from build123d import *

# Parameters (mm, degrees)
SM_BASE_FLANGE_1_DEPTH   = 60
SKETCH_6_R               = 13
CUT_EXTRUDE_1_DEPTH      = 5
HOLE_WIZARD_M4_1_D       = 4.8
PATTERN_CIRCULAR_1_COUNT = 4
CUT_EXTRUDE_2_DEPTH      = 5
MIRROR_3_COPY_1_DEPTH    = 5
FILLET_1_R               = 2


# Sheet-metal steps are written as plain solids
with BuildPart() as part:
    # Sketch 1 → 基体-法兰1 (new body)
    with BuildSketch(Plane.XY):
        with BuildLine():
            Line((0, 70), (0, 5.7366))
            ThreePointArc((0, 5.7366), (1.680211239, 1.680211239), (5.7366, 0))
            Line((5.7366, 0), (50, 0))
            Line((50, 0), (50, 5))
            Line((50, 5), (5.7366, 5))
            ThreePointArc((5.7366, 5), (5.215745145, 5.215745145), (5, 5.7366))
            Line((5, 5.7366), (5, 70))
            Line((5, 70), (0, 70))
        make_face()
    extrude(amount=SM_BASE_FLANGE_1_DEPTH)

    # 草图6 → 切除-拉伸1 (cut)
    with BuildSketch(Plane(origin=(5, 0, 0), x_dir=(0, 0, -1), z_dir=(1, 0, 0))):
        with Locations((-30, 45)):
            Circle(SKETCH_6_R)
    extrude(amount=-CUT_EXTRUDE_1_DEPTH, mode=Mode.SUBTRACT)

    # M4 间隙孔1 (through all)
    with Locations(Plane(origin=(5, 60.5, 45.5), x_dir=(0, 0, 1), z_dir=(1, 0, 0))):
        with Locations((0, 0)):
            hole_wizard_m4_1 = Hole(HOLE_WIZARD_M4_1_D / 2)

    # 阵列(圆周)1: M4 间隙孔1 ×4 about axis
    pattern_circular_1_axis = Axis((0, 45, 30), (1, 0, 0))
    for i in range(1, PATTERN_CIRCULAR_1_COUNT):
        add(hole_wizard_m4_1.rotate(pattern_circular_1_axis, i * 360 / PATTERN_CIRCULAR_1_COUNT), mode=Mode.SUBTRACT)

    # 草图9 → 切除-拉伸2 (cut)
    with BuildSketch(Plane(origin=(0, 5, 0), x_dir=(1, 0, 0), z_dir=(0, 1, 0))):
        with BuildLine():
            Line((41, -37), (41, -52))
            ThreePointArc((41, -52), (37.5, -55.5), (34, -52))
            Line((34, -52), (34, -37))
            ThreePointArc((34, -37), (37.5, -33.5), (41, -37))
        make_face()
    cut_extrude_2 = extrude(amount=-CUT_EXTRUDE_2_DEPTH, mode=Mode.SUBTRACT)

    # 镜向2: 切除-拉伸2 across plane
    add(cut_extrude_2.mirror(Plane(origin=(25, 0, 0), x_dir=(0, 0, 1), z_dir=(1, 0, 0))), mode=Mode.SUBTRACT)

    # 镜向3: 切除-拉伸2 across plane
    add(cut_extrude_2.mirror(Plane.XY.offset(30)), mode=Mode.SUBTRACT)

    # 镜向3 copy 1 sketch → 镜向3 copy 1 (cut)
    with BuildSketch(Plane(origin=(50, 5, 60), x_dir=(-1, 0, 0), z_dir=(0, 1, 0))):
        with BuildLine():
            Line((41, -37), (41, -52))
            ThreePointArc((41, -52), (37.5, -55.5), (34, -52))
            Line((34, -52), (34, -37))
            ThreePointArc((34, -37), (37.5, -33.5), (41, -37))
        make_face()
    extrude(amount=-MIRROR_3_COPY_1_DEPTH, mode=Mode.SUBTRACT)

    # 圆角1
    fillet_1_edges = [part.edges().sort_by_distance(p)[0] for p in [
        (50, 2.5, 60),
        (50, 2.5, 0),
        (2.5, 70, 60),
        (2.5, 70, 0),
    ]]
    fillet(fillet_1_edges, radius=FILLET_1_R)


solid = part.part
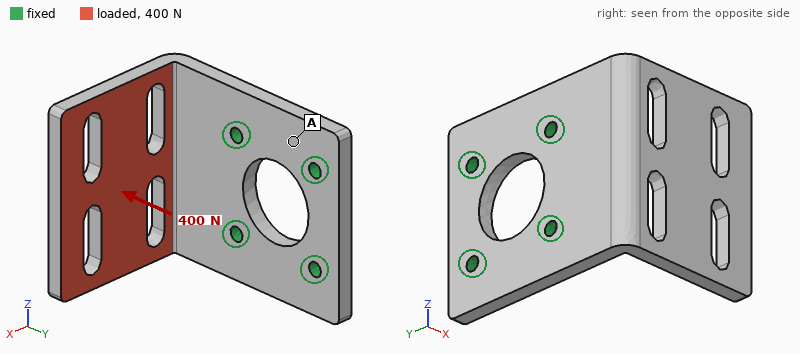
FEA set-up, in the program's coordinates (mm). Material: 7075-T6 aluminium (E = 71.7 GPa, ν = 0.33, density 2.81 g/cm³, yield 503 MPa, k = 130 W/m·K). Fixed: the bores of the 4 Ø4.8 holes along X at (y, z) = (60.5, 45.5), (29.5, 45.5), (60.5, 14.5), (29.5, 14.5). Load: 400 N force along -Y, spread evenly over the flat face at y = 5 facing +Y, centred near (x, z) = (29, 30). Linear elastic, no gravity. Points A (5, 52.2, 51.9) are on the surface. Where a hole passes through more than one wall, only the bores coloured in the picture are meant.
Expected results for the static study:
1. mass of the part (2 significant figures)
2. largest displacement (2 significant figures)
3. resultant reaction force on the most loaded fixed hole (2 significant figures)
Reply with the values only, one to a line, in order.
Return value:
79 g
0.62 mm
190 N
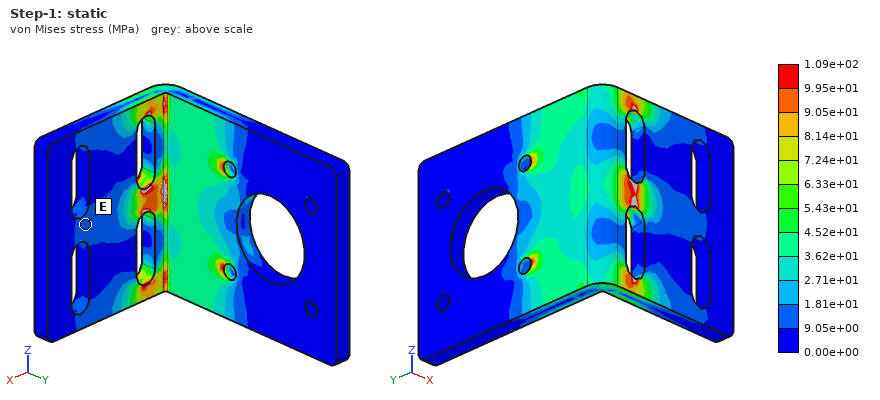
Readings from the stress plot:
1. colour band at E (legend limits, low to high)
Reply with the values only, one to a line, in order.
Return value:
9.05e+00 to 1.81e+01 MPa
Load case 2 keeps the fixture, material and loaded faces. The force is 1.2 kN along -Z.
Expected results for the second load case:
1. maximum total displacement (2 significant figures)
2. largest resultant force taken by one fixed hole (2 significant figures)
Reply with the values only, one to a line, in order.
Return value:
0.39 mm
1.2 kN
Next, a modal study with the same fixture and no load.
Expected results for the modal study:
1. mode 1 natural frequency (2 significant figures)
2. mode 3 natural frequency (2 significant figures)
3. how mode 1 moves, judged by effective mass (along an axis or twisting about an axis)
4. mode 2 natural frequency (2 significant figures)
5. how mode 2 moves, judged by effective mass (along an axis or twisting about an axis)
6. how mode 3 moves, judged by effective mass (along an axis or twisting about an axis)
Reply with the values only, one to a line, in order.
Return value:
890 Hz
2600 Hz
along Y
1800 Hz
along Z
along X
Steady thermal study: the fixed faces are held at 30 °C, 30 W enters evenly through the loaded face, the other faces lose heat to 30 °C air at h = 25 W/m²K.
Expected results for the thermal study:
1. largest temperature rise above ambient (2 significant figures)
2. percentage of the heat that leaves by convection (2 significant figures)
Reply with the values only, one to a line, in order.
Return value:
57 K
19 %
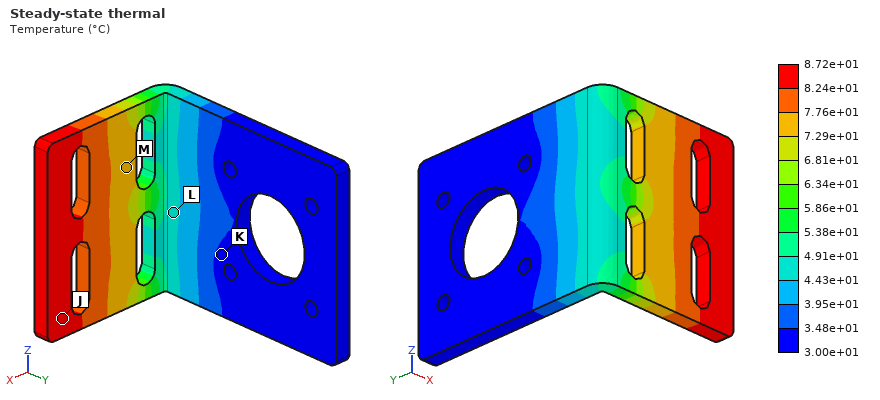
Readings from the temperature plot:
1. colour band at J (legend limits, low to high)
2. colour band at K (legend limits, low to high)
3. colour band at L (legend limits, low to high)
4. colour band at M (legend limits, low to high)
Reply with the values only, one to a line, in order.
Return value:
8.24e+01 to 8.72e+01 °C
3.00e+01 to 3.48e+01 °C
4.43e+01 to 4.91e+01 °C
7.29e+01 to 7.76e+01 °C
